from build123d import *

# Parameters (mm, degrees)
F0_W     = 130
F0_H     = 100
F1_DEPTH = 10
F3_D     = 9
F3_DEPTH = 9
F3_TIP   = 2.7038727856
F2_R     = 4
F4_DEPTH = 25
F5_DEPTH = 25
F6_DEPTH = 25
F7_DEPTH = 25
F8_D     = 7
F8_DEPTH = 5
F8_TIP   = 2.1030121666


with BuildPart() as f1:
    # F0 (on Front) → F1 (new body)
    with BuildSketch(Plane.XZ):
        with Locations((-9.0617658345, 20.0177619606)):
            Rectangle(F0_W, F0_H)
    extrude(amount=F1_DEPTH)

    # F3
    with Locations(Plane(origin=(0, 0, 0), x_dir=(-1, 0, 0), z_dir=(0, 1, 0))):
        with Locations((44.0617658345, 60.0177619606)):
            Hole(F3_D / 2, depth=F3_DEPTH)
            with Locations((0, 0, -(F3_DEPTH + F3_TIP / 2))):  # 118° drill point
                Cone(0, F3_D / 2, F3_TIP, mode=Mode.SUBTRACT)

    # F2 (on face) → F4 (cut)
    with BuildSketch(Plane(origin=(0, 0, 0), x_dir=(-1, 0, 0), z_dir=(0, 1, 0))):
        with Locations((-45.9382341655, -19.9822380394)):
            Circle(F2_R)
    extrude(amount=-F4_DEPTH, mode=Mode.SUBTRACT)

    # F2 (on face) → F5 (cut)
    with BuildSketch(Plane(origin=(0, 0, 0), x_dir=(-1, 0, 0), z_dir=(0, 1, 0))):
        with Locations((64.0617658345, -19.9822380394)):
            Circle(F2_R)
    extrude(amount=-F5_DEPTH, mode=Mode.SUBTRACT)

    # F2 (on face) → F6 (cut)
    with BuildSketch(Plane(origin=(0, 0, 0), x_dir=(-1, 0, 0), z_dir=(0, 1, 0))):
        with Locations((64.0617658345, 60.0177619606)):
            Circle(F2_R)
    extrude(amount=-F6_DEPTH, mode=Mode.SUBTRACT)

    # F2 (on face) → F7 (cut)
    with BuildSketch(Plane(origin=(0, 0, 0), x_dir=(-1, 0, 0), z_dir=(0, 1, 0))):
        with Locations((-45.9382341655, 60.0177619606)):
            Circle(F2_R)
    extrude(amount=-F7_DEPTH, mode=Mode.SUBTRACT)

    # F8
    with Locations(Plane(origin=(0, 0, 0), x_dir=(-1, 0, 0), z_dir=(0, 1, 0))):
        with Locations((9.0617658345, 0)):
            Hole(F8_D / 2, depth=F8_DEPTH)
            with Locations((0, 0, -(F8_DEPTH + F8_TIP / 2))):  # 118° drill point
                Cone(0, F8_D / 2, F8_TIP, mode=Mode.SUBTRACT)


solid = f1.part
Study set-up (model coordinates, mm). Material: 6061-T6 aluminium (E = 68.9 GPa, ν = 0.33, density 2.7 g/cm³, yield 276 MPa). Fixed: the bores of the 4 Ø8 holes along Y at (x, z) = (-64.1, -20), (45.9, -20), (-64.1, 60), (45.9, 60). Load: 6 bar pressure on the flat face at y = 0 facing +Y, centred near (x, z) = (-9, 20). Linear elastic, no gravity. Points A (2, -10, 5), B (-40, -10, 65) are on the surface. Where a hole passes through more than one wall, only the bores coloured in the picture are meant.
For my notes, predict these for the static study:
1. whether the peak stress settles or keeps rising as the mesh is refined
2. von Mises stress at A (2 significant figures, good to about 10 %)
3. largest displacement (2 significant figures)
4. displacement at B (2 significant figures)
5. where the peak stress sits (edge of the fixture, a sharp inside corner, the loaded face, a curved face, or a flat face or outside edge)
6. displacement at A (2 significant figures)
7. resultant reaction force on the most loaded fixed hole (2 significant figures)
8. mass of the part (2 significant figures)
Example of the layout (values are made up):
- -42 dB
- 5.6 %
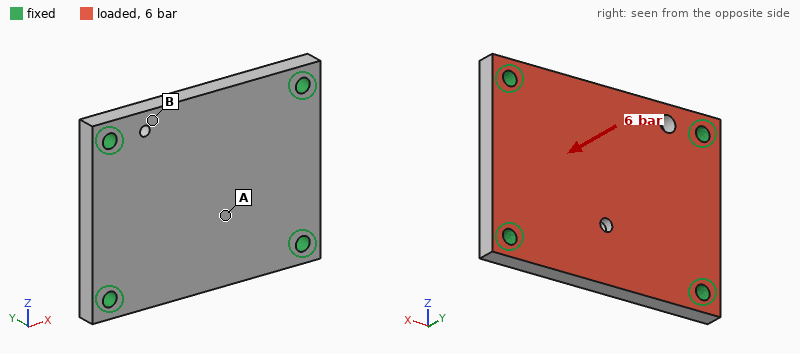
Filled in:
- keeps rising
- 17 MPa
- 66 µm
- 27 µm
- edge of the fixture
- 61 µm
- 1.9 kN
- 340 g
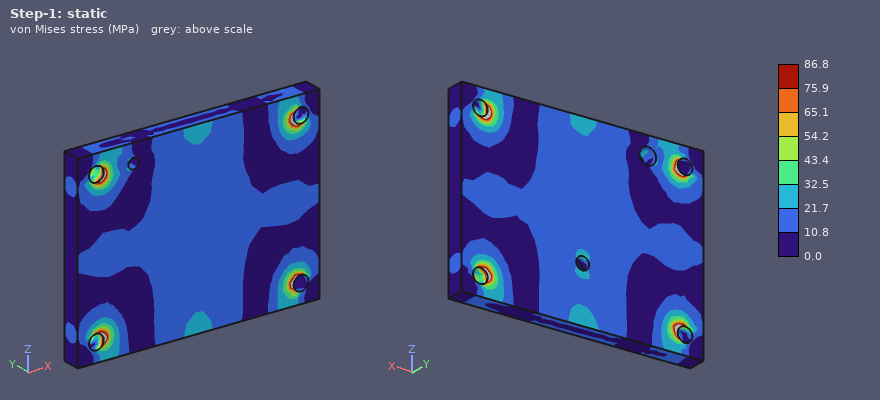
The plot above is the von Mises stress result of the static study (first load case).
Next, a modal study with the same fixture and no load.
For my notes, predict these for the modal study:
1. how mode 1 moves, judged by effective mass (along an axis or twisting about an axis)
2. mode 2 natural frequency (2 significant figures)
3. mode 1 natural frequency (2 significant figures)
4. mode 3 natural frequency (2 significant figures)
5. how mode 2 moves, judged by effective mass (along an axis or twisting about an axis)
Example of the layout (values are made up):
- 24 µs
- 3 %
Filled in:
- along Y
- 5100 Hz
- 3400 Hz
- 7200 Hz
- twisting about X
